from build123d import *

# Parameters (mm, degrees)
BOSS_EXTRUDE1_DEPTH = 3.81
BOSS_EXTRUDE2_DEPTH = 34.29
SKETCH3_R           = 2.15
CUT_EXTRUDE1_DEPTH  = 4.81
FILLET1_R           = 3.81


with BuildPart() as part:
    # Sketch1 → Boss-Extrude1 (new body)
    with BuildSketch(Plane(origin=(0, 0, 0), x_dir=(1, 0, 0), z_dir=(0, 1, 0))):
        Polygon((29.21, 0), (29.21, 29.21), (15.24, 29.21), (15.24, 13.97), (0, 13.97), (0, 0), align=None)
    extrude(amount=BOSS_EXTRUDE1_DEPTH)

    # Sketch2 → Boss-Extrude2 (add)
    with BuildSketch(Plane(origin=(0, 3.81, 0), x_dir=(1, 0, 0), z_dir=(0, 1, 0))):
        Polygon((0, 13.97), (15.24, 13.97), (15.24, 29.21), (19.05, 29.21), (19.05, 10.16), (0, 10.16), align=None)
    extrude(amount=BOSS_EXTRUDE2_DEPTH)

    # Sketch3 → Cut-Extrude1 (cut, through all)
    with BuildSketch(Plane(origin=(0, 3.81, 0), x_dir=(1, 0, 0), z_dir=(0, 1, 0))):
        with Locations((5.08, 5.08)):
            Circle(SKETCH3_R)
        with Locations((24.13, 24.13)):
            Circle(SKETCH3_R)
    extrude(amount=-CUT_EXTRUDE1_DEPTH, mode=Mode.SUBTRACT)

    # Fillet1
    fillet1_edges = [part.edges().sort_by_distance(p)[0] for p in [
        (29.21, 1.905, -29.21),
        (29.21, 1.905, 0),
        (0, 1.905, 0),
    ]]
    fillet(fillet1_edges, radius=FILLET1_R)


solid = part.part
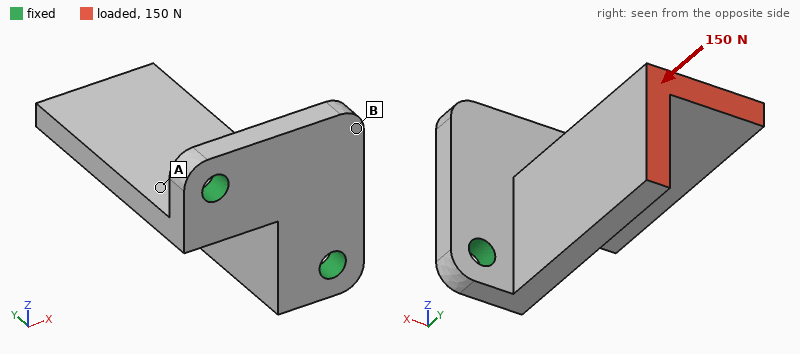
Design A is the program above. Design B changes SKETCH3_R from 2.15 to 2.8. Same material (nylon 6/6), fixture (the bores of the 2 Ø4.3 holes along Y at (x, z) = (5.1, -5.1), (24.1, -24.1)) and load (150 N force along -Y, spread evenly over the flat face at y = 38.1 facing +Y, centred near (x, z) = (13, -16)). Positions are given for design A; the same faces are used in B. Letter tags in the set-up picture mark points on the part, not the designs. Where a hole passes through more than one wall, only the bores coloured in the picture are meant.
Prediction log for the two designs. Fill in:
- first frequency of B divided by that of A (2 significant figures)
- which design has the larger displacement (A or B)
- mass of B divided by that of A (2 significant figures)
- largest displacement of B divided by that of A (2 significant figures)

1.1
A
0.99
0.73
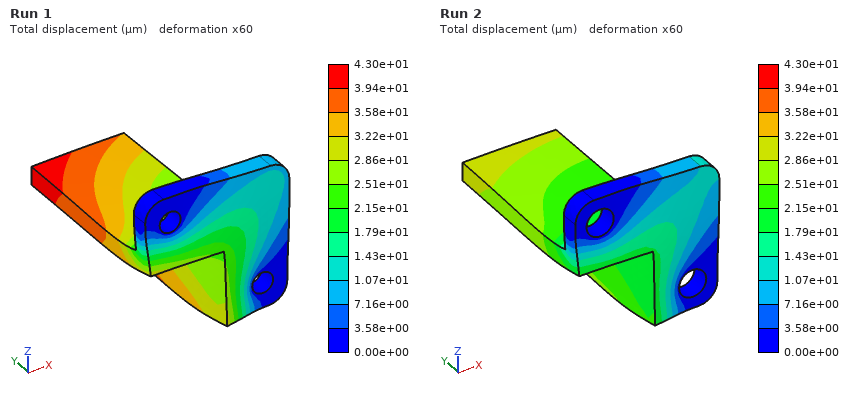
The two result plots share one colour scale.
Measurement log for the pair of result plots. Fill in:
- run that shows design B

Run 2
